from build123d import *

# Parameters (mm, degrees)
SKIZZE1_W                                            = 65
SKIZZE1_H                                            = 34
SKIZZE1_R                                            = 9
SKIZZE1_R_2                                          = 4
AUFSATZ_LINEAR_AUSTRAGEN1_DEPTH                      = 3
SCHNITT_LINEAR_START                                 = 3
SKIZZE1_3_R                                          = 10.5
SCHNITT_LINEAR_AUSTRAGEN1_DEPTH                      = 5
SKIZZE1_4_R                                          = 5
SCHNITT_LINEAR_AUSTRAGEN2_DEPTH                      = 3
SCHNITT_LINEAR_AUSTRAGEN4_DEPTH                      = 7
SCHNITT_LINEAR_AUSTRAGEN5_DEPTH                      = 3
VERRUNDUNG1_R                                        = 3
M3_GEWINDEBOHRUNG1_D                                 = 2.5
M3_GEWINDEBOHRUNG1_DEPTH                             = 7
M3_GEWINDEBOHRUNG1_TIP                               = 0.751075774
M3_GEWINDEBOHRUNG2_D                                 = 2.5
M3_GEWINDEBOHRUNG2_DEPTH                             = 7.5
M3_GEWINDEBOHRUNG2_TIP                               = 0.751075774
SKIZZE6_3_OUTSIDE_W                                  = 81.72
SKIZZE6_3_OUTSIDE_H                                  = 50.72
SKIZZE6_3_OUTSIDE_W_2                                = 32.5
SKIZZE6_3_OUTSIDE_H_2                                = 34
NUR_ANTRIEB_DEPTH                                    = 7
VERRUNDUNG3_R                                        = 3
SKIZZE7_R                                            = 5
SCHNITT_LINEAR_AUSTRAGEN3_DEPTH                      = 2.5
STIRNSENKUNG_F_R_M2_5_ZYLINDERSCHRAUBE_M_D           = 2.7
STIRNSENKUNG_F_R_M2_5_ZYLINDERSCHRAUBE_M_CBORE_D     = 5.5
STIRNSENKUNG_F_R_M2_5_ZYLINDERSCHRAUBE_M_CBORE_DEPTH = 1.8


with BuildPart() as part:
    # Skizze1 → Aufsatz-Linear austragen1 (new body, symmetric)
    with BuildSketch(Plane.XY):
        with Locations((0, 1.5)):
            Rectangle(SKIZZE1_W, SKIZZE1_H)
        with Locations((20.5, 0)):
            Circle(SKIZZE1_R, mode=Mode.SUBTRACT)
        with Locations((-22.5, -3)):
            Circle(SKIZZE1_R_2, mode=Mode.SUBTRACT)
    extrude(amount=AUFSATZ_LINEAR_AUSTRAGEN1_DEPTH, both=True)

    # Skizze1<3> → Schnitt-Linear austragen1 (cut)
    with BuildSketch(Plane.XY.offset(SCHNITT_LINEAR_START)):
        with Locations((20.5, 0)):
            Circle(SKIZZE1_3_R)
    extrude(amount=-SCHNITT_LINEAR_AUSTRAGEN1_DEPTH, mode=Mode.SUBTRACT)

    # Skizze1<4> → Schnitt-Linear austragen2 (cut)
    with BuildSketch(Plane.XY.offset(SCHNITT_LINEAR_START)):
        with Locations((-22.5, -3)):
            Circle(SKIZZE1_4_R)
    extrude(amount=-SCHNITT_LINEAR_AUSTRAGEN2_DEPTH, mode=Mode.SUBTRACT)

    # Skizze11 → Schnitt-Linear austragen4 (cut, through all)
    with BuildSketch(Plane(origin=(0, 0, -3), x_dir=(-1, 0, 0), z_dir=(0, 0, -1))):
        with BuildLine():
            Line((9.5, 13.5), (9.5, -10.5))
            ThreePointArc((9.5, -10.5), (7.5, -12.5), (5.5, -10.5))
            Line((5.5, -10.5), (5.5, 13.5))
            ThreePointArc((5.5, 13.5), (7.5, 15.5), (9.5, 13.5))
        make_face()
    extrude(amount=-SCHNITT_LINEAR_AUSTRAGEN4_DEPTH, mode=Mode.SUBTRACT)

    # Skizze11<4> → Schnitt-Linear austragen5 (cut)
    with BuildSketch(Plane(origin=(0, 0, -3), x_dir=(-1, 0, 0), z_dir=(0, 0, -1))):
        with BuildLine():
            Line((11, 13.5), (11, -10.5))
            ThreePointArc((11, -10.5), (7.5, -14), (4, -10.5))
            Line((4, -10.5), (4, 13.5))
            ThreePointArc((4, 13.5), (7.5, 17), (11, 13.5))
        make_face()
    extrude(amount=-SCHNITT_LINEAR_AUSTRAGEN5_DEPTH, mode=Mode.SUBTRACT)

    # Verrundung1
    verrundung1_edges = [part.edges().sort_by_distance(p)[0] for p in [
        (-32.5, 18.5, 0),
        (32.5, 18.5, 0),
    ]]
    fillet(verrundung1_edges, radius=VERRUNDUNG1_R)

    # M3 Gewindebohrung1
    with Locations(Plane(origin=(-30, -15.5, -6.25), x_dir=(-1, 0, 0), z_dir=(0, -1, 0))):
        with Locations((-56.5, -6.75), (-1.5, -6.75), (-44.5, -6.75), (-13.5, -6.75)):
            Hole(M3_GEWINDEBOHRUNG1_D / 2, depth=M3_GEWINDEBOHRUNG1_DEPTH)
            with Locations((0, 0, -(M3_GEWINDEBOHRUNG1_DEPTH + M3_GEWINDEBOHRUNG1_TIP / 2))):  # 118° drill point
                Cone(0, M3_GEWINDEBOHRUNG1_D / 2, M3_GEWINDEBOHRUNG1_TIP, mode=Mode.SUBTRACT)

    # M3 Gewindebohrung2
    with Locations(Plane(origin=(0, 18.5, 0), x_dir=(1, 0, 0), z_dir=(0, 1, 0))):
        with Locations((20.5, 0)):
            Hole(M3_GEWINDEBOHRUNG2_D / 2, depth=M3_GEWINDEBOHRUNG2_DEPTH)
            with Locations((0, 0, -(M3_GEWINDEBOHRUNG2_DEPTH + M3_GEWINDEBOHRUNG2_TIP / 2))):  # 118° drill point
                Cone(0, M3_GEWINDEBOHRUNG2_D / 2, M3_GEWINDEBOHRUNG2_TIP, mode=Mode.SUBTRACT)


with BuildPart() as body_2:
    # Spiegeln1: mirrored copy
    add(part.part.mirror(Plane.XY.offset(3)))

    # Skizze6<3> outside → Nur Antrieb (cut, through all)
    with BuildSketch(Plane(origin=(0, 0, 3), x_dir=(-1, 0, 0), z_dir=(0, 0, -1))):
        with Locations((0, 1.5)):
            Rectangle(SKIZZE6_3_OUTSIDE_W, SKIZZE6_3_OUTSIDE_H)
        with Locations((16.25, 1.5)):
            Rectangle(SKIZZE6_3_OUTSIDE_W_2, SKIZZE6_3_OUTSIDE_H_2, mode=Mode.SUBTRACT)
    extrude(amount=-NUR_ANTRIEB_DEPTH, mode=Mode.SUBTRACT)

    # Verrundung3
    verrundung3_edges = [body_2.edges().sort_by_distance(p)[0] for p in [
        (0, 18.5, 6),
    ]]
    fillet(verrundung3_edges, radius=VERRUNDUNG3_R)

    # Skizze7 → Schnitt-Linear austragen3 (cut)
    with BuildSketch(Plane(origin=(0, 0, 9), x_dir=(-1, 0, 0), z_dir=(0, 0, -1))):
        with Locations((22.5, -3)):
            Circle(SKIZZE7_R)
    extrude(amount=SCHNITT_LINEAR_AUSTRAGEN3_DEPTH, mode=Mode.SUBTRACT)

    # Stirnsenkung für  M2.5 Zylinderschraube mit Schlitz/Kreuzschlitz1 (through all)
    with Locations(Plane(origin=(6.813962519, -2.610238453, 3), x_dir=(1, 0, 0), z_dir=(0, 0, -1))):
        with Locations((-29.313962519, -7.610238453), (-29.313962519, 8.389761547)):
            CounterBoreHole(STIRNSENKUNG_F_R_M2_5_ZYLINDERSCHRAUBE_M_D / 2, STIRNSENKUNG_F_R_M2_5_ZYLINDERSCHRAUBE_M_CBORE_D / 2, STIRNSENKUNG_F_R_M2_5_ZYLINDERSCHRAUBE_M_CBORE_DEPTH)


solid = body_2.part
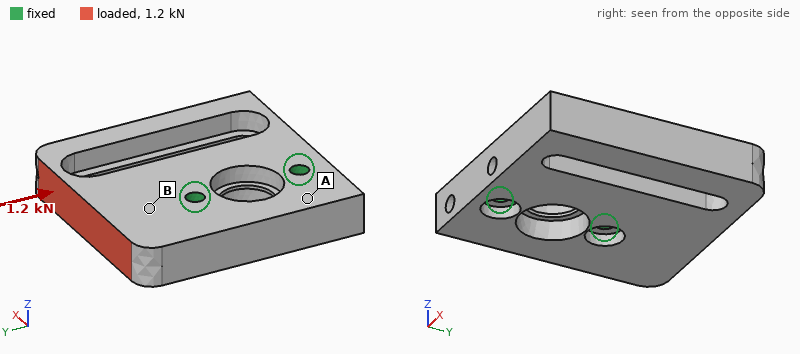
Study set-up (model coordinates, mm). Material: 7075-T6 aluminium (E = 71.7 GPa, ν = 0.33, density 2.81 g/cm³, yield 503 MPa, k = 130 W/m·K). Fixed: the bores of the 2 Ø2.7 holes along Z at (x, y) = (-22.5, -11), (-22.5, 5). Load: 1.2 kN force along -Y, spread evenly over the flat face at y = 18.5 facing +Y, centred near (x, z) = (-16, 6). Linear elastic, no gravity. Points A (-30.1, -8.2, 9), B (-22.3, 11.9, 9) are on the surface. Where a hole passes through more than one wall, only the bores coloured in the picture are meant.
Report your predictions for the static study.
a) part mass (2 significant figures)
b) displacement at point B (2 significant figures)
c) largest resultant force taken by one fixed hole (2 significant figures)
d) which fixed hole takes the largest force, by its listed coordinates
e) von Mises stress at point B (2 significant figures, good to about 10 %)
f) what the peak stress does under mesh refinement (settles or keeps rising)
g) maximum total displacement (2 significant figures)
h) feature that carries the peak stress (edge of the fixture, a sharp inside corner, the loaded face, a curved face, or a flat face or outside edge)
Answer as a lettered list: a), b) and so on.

a) 14 g
b) 3.1 µm
c) 970 N
d) (-22.5, 5)
e) 13 MPa
f) keeps rising
g) 19 µm
h) edge of the fixture
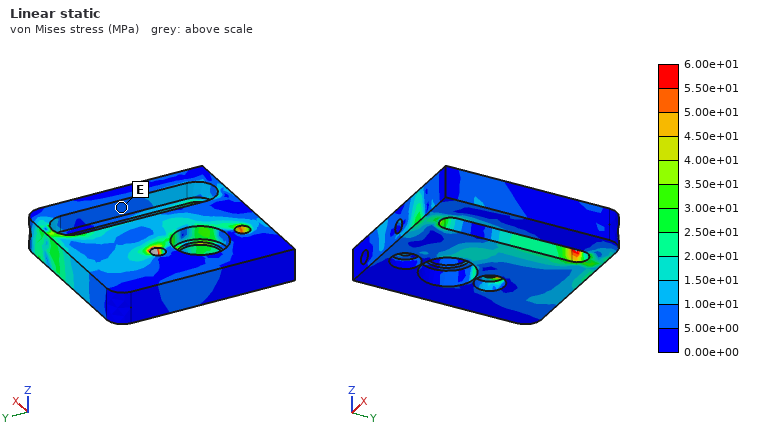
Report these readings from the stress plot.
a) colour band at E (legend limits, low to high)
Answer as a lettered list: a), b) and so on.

a) 5.00e+00 to 1.00e+01 MPa
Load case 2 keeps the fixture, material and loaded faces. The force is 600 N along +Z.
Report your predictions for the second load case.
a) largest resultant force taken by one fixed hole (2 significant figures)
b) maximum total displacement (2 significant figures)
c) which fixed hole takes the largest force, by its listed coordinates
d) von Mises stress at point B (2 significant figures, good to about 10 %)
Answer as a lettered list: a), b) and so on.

a) 870 N
b) 92 µm
c) (-22.5, 5)
d) 36 MPa
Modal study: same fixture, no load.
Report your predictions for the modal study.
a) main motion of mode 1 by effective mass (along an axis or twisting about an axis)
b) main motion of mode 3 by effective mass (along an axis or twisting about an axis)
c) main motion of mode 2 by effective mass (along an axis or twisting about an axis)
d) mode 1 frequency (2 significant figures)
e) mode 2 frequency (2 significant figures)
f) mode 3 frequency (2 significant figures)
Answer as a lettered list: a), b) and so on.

a) along Z
b) along Y
c) twisting about X
d) 5500 Hz
e) 10 kHz
f) 12 kHz
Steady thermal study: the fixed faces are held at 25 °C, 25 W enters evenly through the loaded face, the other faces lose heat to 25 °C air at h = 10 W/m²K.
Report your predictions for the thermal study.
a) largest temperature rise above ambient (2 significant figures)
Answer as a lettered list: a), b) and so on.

a) 36 K
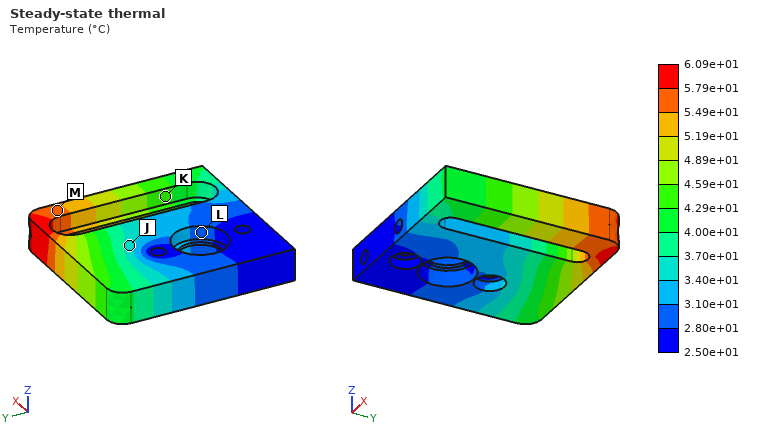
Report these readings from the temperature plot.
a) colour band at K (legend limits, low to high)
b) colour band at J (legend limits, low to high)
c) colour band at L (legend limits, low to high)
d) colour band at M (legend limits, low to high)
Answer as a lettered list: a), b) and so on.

a) 4.29e+01 to 4.59e+01 °C
b) 3.40e+01 to 3.70e+01 °C
c) 2.80e+01 to 3.10e+01 °C
d) 5.49e+01 to 5.79e+01 °C
